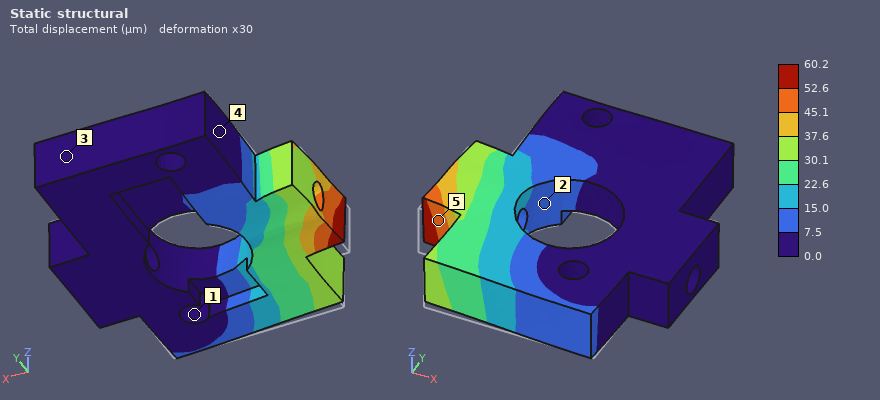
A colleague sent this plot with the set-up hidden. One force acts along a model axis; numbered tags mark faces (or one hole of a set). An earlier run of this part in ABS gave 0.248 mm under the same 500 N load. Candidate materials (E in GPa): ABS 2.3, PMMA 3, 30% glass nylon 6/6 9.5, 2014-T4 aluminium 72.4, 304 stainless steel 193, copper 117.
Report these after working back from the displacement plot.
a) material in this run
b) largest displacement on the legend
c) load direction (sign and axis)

30% glass nylon 6/6
60.2 µm
+Y
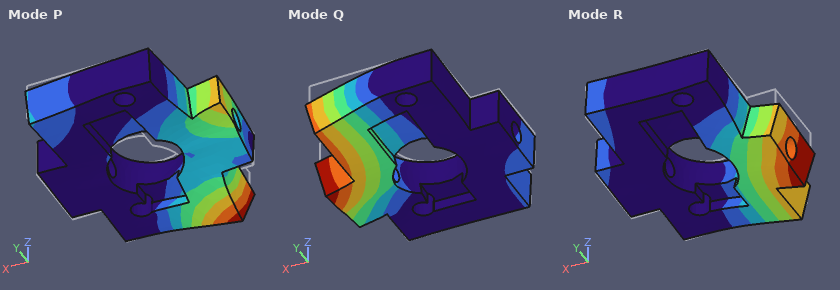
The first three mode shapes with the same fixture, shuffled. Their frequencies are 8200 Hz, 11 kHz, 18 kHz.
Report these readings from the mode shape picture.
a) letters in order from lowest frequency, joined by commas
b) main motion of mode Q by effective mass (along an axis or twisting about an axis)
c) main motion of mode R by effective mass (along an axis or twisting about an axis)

R, Q, P
along Z
along Z
